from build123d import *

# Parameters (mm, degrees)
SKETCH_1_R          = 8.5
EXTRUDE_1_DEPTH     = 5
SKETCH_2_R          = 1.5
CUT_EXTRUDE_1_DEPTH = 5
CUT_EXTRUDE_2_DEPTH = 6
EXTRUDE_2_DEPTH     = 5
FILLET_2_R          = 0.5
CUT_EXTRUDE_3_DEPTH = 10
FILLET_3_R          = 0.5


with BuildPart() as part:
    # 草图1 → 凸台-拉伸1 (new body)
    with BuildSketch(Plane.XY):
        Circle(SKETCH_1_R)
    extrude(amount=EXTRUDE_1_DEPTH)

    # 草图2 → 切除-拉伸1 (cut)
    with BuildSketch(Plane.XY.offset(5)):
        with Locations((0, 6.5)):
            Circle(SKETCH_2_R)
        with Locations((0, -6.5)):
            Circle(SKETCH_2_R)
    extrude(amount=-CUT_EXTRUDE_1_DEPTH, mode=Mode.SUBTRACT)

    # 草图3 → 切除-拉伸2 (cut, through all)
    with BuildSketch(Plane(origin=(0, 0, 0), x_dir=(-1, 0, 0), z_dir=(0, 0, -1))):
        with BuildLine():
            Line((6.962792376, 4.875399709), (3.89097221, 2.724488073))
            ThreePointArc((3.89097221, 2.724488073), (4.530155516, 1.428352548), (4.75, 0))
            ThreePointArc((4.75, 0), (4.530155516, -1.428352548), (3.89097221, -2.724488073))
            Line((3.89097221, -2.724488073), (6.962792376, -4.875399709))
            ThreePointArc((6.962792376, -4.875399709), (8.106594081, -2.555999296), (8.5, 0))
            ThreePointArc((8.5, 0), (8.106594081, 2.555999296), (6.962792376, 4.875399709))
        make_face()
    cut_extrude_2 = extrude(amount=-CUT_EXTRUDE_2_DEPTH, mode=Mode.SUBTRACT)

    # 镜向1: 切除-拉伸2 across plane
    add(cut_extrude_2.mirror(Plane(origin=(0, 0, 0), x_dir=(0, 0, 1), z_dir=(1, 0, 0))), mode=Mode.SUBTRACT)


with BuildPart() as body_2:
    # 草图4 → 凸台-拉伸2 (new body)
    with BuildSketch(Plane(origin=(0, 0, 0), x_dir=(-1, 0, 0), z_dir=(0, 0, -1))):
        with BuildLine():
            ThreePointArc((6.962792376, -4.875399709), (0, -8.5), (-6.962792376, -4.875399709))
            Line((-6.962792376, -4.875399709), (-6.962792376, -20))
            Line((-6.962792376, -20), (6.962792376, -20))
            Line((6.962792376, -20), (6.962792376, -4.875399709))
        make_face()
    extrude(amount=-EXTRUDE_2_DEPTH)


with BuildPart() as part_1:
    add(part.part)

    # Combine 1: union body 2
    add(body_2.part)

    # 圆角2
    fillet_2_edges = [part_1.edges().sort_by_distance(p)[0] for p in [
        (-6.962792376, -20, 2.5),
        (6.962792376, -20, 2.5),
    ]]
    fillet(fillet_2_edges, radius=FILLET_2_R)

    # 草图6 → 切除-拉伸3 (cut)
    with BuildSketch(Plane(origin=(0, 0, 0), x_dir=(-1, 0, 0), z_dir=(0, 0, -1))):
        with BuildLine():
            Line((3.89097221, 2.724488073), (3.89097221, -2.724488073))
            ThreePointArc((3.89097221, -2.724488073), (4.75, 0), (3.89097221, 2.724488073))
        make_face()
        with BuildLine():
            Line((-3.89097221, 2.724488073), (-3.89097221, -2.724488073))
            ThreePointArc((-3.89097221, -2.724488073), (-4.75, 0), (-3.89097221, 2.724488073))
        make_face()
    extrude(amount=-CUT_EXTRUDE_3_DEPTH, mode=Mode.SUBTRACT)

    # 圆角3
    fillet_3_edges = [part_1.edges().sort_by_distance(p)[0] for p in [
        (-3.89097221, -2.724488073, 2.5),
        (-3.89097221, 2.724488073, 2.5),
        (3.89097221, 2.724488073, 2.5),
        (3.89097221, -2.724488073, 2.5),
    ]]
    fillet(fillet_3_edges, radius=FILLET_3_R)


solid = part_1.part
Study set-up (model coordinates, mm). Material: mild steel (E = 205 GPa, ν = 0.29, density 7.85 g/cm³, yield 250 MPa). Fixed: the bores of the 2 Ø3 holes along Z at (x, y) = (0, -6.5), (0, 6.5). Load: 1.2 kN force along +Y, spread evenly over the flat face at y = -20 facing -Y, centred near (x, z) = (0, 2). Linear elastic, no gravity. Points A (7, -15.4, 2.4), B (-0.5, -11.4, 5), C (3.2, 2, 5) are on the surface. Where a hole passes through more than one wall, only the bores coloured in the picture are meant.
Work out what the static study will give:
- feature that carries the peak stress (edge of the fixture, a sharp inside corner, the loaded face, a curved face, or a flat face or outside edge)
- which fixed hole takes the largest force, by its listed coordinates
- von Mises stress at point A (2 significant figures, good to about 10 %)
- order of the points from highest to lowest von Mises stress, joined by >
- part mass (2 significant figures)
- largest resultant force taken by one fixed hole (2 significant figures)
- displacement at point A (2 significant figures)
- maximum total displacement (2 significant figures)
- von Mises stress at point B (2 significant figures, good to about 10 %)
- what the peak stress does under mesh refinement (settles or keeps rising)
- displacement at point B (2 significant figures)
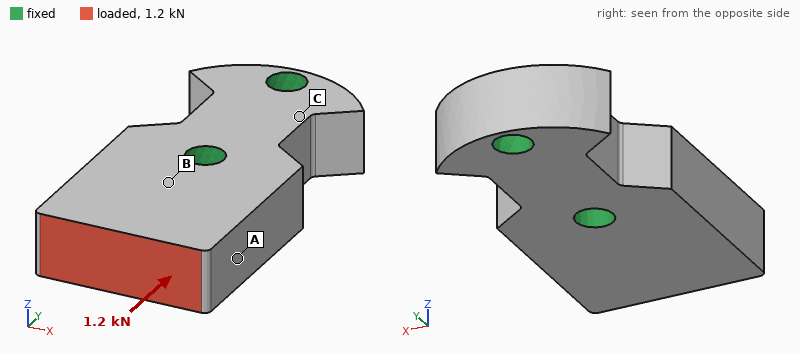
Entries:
edge of the fixture
(0, -6.5)
13 MPa
B > A > C
13 g
1.1 kN
0.99 µm
1.4 µm
27 MPa
keeps rising
0.55 µm
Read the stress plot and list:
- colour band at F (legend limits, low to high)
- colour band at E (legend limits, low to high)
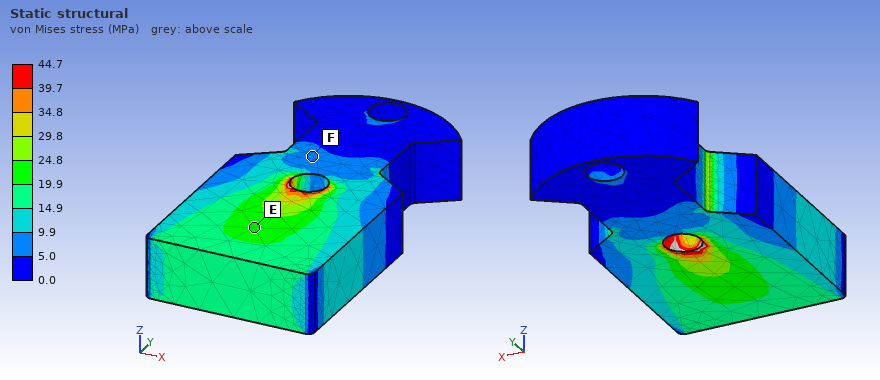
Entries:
5.0 to 9.9 MPa
19.9 to 24.8 MPa
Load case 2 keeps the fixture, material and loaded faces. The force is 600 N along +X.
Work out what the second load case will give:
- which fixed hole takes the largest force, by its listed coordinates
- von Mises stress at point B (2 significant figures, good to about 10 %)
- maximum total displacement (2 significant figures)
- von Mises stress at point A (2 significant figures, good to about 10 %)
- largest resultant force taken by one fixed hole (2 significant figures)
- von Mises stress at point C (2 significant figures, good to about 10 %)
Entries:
(0, -6.5)
26 MPa
9.8 µm
19 MPa
930 N
17 MPa
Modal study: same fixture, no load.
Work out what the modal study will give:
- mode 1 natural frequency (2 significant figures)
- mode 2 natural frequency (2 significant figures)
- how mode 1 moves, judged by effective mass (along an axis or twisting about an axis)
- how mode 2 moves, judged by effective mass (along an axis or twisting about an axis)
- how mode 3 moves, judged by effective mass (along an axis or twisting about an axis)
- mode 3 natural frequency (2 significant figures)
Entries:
20 kHz
25 kHz
along Z
along X
twisting about Y
34 kHz
